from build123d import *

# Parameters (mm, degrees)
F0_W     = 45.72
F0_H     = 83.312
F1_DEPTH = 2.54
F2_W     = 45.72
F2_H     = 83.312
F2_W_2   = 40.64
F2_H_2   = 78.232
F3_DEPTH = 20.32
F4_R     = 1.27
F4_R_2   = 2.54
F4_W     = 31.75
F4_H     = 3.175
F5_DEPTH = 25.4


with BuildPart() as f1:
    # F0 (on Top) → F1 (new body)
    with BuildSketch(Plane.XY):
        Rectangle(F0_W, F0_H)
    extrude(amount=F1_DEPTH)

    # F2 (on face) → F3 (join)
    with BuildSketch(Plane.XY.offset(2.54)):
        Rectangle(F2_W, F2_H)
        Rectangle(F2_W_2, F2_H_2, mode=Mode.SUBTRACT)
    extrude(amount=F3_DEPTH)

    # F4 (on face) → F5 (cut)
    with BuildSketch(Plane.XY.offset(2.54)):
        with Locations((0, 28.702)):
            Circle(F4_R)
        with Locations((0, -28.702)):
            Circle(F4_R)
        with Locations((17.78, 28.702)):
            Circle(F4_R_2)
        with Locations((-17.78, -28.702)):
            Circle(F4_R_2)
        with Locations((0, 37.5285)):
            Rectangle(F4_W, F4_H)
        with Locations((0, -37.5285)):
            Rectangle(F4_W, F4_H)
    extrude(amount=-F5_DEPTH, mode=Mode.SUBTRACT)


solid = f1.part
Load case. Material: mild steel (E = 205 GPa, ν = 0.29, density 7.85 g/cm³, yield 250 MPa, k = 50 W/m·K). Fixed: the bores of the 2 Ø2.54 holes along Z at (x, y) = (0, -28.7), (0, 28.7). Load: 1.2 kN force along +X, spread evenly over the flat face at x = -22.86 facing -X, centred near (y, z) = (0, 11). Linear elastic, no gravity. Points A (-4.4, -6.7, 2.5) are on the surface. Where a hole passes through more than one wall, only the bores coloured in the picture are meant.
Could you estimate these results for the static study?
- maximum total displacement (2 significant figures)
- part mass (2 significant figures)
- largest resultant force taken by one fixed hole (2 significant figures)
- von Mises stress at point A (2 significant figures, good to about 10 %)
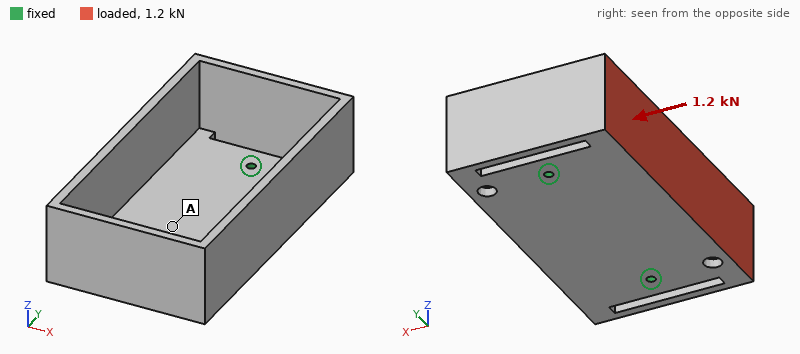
0.24 mm
170 g
600 N
35 MPa
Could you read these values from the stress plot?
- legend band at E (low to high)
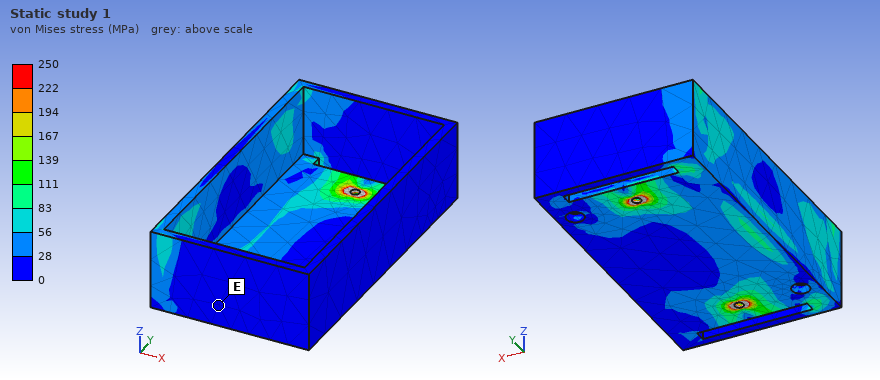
0 to 28 MPa
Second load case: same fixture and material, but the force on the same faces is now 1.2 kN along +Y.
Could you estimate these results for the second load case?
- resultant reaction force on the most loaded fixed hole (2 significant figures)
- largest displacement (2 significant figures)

790 N
72 µm
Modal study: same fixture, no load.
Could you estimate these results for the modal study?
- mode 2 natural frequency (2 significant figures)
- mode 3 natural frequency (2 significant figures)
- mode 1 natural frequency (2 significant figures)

1800 Hz
2100 Hz
1000 Hz
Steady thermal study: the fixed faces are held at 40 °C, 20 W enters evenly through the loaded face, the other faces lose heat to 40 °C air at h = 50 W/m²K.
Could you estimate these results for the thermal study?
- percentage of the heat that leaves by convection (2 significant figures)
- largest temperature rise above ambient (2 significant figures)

65 %
44 K
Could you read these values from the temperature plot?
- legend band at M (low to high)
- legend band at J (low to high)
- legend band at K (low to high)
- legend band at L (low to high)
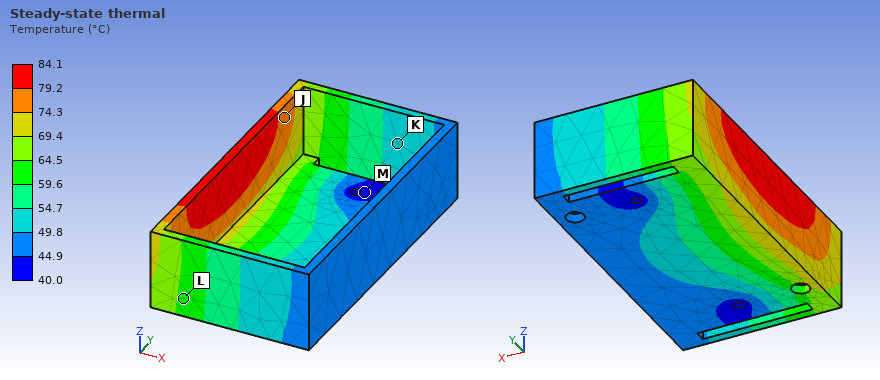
40.0 to 44.9 °C
74.3 to 79.2 °C
49.8 to 54.7 °C
59.6 to 64.5 °C
